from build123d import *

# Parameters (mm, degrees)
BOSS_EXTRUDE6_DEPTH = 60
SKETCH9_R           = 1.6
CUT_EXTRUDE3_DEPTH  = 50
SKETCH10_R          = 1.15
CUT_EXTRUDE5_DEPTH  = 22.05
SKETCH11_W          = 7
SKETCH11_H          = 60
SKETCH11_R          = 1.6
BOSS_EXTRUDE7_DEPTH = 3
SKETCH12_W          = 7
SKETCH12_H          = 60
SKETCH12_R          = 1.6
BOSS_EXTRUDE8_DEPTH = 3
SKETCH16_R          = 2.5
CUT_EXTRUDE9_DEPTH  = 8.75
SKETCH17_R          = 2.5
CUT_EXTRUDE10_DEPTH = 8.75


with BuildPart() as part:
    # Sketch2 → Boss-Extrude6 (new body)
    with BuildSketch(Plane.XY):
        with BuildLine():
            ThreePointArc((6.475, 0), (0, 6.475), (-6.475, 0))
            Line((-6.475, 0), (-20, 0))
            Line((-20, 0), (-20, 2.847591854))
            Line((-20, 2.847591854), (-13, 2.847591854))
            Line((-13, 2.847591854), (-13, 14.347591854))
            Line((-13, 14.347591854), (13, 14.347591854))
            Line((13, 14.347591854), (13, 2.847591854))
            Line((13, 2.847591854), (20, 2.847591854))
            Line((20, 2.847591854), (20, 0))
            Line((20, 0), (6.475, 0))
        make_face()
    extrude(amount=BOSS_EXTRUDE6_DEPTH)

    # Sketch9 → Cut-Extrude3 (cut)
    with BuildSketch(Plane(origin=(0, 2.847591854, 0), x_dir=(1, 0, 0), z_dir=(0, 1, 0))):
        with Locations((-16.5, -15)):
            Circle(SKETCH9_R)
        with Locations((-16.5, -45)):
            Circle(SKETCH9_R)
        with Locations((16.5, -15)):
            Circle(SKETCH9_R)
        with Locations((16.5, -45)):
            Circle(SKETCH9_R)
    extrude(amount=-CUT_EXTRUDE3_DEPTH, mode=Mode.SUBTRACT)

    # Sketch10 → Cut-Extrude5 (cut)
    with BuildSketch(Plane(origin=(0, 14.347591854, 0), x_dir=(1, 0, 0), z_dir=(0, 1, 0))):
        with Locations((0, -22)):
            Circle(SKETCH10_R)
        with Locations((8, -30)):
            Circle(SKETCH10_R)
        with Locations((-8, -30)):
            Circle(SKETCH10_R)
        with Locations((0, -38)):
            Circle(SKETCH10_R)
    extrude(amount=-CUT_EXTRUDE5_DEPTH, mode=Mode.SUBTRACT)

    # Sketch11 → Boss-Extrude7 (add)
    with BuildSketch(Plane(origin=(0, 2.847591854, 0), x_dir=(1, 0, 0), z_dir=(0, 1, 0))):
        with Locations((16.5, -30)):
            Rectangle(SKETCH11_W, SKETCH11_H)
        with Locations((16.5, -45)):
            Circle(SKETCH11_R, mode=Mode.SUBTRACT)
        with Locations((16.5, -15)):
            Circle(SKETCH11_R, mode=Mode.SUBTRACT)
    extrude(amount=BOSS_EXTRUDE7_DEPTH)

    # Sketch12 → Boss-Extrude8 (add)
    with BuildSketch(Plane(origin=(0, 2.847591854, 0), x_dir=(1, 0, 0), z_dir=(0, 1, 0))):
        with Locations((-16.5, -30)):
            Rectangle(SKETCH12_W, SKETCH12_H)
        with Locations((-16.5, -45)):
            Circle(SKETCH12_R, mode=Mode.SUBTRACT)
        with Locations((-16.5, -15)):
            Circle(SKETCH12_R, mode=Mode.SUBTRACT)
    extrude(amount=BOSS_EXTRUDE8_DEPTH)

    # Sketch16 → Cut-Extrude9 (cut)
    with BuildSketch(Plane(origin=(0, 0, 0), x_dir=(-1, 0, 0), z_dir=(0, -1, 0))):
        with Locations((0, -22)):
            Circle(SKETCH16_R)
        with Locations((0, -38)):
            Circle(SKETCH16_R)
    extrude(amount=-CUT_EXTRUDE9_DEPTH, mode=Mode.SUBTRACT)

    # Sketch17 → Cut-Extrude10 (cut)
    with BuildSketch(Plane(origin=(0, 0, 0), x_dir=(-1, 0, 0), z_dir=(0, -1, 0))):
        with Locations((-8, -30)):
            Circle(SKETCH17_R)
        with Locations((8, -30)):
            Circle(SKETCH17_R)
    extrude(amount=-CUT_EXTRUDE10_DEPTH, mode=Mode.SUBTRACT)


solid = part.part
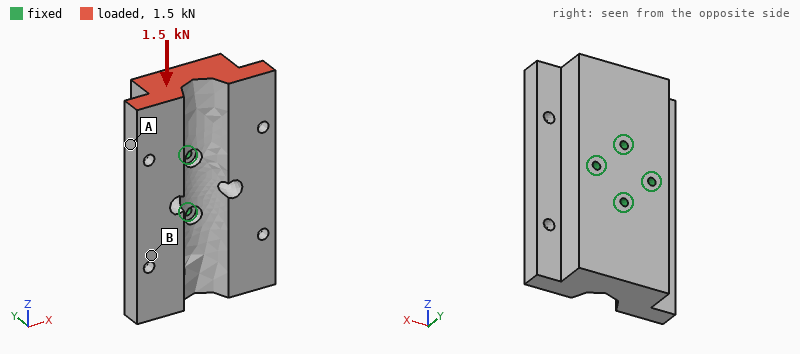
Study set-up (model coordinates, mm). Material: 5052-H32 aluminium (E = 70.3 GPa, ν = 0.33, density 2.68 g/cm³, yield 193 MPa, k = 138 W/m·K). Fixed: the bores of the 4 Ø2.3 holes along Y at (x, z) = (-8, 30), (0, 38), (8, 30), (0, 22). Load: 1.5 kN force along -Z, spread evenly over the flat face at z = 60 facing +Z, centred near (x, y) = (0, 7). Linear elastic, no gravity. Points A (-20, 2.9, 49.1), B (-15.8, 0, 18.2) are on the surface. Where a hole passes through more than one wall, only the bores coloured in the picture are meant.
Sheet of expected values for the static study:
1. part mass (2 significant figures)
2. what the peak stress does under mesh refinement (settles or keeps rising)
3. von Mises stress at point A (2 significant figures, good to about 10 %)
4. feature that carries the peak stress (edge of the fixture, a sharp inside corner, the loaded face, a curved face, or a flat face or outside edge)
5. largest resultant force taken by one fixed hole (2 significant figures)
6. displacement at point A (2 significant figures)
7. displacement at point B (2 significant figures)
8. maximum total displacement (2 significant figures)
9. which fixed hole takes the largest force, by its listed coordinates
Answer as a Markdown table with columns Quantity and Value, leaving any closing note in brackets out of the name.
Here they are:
| Quantity | Value |
|---|---|
| part mass | 61 g |
| what the peak stress does under mesh refinement | keeps rising |
| von Mises stress at point A | 4.8 MPa |
| feature that carries the peak stress | edge of the fixture |
| largest resultant force taken by one fixed hole | 580 N |
| displacement at point A | 4.2 µm |
| displacement at point B | 2.4 µm |
| maximum total displacement | 6.5 µm |
| which fixed hole takes the largest force, by its listed coordinates | (0, 38) |
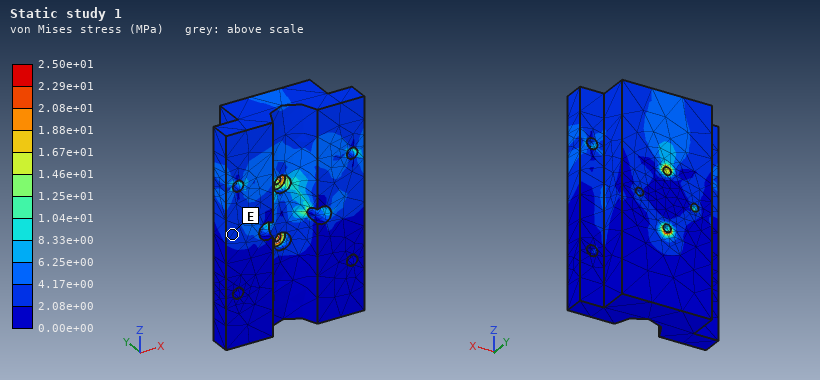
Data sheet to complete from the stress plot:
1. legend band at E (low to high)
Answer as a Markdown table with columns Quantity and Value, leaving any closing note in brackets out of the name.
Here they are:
| Quantity | Value |
|---|---|
| legend band at E | 2.08e+00 to 4.17e+00 MPa |
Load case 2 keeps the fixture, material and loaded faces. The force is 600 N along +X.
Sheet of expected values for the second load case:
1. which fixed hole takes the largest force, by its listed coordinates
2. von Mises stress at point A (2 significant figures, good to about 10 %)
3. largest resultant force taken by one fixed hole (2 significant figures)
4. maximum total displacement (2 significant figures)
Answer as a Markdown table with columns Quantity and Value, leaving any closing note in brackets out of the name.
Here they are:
| Quantity | Value |
|---|---|
| which fixed hole takes the largest force, by its listed coordinates | (0, 38) |
| von Mises stress at point A | 5.0 MPa |
| largest resultant force taken by one fixed hole | 740 N |
| maximum total displacement | 11 µm |
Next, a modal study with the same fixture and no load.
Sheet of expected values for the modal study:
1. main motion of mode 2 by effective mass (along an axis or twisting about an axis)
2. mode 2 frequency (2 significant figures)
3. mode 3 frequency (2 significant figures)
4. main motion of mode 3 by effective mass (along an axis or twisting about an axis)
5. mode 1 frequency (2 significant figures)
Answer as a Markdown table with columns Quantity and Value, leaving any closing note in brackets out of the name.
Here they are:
| Quantity | Value |
|---|---|
| main motion of mode 2 by effective mass | along X |
| mode 2 frequency | 10 kHz |
| mode 3 frequency | 11 kHz |
| main motion of mode 3 by effective mass | twisting about Y |
| mode 1 frequency | 7600 Hz |
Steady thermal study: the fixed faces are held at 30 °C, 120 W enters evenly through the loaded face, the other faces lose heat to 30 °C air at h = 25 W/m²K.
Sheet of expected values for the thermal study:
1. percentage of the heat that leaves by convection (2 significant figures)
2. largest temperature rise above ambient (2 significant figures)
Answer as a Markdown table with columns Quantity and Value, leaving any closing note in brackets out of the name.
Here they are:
| Quantity | Value |
|---|---|
| percentage of the heat that leaves by convection | 3.2 % |
| largest temperature rise above ambient | 69 K |
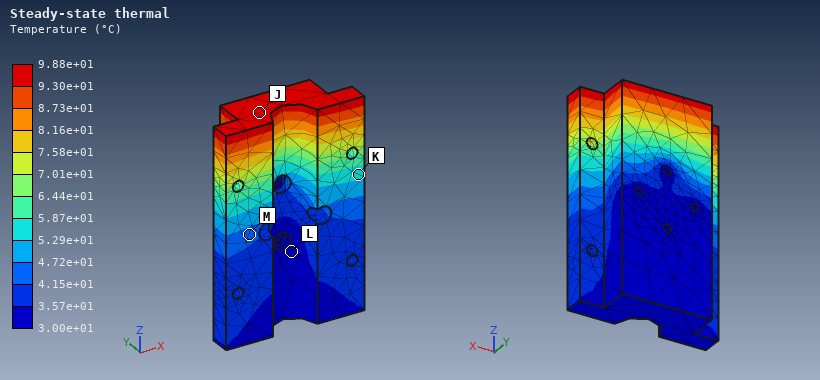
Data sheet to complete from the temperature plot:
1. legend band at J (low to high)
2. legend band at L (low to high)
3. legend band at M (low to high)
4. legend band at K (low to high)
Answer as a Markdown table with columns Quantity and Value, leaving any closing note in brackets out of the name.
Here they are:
| Quantity | Value |
|---|---|
| legend band at J | 9.30e+01 to 9.88e+01 °C |
| legend band at L | 3.00e+01 to 3.57e+01 °C |
| legend band at M | 4.15e+01 to 4.72e+01 °C |
| legend band at K | 5.29e+01 to 5.87e+01 °C |
